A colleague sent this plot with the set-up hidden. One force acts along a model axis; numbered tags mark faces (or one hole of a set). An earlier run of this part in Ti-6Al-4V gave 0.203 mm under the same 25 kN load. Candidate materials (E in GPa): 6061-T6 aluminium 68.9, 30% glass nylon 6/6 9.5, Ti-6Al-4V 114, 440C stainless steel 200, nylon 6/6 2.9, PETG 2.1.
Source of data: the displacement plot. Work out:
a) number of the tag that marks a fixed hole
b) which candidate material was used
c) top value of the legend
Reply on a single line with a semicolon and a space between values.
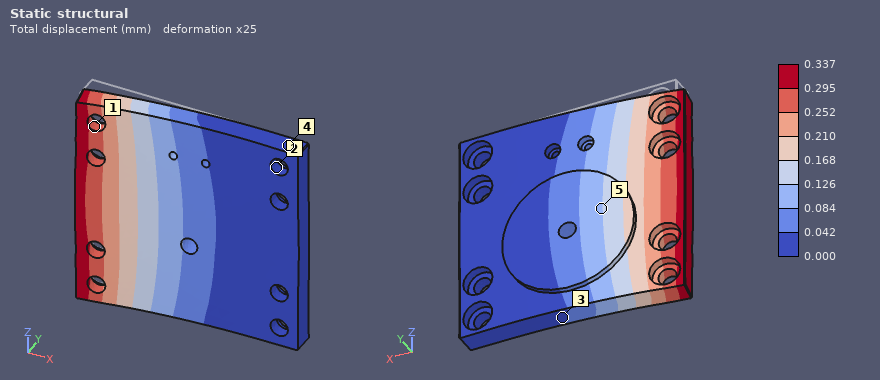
2; 6061-T6 aluminium; 0.337 mm
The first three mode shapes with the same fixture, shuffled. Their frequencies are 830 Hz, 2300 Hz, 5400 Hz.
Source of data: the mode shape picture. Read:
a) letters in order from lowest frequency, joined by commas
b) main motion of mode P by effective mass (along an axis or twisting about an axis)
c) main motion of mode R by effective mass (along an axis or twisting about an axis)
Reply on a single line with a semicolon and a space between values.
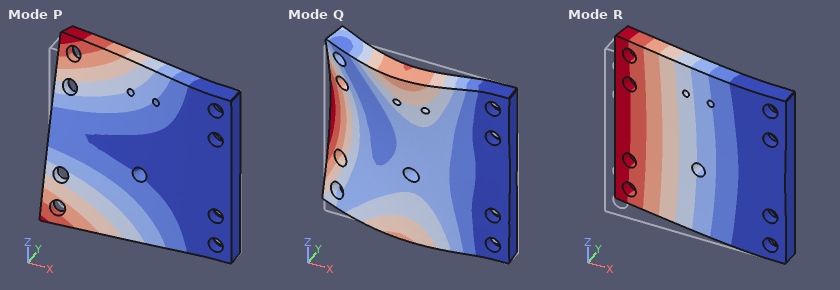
R, P, Q; twisting about X; along Y
